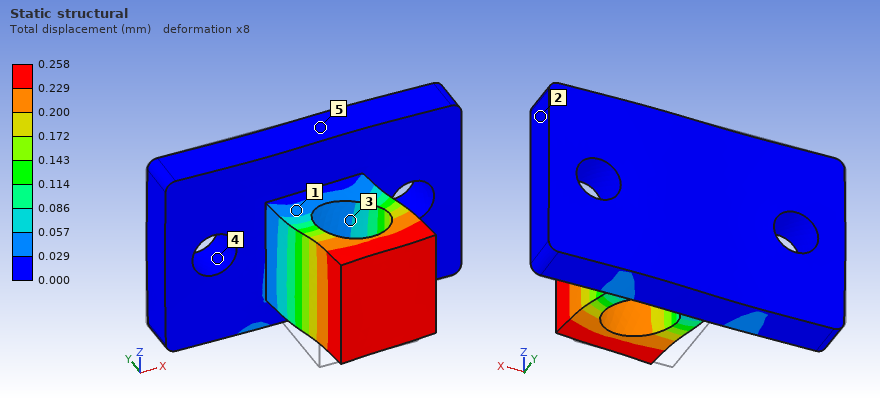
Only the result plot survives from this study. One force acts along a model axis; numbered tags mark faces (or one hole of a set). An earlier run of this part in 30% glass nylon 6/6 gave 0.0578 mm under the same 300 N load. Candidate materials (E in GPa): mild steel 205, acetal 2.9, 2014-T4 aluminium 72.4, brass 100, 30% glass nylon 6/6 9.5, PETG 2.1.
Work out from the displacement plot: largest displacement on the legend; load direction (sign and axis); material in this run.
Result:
0.258 mm
+X
PETG
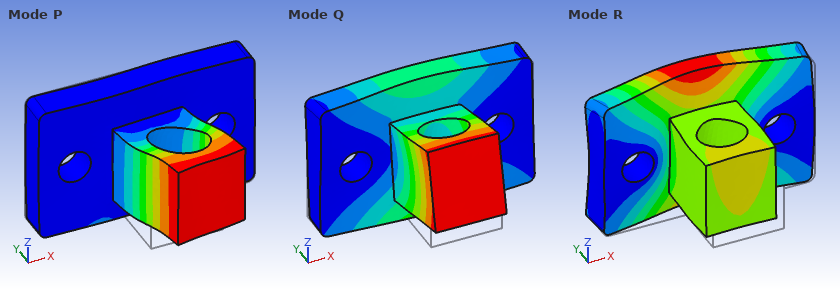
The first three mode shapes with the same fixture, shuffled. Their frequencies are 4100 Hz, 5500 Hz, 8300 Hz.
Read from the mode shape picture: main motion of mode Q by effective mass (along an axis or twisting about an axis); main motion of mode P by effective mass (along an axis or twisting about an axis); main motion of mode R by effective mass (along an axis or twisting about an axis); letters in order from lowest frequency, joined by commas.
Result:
along Z
along X
along Y
Q, P, R
